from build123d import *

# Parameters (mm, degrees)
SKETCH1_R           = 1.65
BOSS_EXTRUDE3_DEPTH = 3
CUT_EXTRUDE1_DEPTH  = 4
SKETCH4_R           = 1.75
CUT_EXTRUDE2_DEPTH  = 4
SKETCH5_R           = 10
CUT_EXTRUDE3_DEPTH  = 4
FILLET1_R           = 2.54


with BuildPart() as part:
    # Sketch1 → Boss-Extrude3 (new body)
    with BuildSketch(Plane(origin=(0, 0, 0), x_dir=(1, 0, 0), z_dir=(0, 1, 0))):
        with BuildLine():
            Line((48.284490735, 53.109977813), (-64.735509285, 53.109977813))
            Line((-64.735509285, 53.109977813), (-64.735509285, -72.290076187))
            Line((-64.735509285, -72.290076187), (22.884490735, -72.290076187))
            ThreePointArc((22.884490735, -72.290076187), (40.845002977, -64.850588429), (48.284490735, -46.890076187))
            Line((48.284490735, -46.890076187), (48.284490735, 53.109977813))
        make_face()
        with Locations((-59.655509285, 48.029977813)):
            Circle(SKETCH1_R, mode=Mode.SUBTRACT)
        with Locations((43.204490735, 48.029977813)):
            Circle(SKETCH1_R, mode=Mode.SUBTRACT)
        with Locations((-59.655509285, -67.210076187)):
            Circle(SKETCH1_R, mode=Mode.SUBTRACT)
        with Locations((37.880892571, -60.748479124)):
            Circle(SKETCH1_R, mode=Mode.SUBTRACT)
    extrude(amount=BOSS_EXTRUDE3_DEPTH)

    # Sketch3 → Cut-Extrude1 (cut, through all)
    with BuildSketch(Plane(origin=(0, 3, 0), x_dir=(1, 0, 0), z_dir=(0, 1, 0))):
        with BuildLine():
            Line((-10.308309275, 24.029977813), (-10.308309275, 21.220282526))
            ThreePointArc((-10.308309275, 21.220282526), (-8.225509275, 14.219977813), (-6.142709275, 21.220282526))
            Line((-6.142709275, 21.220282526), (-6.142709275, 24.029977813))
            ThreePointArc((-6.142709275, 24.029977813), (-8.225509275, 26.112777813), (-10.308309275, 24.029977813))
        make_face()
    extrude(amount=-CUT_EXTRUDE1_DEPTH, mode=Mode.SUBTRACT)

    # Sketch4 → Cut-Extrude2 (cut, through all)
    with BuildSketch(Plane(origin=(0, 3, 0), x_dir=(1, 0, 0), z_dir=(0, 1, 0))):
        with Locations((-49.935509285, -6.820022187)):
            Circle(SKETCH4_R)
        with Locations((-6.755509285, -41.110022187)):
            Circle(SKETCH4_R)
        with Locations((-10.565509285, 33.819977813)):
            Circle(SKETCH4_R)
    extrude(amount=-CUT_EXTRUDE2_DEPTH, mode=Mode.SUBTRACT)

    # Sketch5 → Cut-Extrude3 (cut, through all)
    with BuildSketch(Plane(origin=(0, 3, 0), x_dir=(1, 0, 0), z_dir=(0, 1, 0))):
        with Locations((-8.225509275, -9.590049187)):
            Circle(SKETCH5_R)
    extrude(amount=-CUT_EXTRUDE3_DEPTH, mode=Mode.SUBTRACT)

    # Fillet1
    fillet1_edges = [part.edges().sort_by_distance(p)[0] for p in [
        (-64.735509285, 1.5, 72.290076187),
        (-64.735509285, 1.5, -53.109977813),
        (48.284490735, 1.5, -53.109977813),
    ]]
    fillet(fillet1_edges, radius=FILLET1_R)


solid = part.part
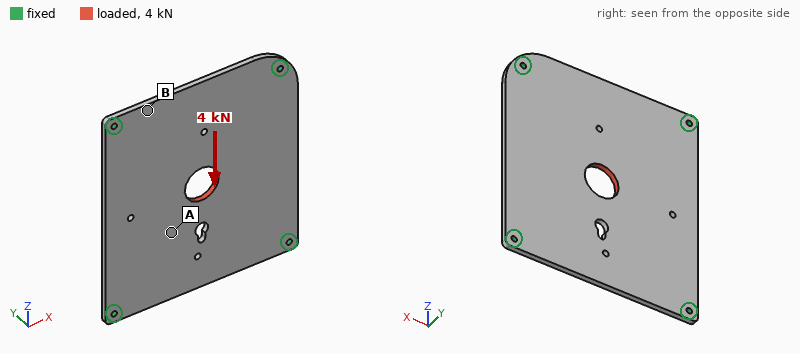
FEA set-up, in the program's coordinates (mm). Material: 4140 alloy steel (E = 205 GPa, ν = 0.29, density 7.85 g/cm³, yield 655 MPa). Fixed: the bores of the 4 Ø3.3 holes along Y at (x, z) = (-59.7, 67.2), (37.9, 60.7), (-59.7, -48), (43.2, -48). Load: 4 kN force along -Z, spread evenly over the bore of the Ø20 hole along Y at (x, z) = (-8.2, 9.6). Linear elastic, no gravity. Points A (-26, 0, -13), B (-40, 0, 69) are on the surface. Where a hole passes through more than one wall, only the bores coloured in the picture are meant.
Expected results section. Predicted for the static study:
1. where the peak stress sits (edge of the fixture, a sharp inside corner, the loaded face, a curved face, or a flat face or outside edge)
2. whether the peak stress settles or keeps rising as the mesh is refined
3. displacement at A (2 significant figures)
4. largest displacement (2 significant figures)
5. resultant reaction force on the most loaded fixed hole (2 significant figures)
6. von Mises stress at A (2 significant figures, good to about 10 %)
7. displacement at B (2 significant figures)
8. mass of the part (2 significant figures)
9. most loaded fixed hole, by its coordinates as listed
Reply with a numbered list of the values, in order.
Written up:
1. edge of the fixture
2. keeps rising
3. 4.7 µm
4. 6.7 µm
5. 1.2 kN
6. 12 MPa
7. 3.3 µm
8. 320 g
9. (37.9, 60.7)
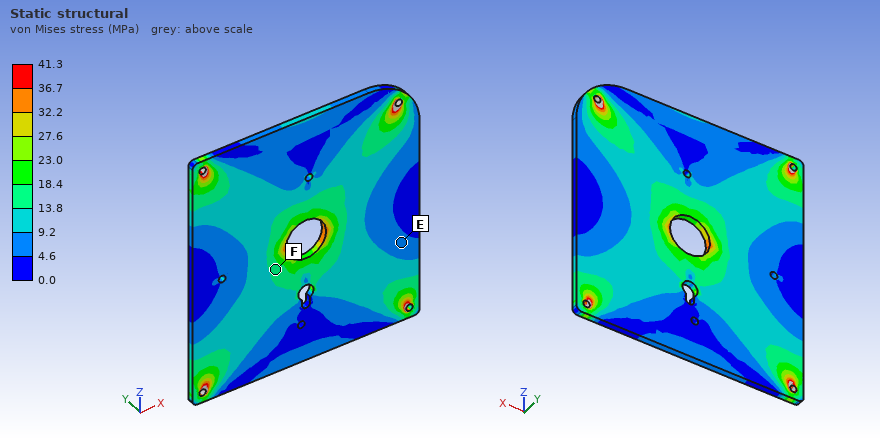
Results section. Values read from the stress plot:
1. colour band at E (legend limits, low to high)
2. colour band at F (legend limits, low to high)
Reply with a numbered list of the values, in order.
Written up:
1. 4.6 to 9.2 MPa
2. 13.8 to 18.4 MPa
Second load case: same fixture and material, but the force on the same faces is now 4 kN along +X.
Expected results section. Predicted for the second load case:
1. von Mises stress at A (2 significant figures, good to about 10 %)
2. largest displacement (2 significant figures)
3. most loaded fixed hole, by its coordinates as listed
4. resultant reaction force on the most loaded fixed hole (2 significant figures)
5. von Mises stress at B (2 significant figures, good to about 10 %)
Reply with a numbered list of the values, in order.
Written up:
1. 14 MPa
2. 7.5 µm
3. (37.9, 60.7)
4. 1.3 kN
5. 11 MPa
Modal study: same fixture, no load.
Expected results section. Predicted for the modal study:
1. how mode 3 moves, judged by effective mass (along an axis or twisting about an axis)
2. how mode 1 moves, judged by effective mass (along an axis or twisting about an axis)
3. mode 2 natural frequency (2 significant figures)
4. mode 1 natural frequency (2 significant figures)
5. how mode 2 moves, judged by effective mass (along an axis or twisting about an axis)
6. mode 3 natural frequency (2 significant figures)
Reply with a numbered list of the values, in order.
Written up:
1. twisting about X
2. along Y
3. 1400 Hz
4. 810 Hz
5. twisting about Z
6. 1600 Hz
